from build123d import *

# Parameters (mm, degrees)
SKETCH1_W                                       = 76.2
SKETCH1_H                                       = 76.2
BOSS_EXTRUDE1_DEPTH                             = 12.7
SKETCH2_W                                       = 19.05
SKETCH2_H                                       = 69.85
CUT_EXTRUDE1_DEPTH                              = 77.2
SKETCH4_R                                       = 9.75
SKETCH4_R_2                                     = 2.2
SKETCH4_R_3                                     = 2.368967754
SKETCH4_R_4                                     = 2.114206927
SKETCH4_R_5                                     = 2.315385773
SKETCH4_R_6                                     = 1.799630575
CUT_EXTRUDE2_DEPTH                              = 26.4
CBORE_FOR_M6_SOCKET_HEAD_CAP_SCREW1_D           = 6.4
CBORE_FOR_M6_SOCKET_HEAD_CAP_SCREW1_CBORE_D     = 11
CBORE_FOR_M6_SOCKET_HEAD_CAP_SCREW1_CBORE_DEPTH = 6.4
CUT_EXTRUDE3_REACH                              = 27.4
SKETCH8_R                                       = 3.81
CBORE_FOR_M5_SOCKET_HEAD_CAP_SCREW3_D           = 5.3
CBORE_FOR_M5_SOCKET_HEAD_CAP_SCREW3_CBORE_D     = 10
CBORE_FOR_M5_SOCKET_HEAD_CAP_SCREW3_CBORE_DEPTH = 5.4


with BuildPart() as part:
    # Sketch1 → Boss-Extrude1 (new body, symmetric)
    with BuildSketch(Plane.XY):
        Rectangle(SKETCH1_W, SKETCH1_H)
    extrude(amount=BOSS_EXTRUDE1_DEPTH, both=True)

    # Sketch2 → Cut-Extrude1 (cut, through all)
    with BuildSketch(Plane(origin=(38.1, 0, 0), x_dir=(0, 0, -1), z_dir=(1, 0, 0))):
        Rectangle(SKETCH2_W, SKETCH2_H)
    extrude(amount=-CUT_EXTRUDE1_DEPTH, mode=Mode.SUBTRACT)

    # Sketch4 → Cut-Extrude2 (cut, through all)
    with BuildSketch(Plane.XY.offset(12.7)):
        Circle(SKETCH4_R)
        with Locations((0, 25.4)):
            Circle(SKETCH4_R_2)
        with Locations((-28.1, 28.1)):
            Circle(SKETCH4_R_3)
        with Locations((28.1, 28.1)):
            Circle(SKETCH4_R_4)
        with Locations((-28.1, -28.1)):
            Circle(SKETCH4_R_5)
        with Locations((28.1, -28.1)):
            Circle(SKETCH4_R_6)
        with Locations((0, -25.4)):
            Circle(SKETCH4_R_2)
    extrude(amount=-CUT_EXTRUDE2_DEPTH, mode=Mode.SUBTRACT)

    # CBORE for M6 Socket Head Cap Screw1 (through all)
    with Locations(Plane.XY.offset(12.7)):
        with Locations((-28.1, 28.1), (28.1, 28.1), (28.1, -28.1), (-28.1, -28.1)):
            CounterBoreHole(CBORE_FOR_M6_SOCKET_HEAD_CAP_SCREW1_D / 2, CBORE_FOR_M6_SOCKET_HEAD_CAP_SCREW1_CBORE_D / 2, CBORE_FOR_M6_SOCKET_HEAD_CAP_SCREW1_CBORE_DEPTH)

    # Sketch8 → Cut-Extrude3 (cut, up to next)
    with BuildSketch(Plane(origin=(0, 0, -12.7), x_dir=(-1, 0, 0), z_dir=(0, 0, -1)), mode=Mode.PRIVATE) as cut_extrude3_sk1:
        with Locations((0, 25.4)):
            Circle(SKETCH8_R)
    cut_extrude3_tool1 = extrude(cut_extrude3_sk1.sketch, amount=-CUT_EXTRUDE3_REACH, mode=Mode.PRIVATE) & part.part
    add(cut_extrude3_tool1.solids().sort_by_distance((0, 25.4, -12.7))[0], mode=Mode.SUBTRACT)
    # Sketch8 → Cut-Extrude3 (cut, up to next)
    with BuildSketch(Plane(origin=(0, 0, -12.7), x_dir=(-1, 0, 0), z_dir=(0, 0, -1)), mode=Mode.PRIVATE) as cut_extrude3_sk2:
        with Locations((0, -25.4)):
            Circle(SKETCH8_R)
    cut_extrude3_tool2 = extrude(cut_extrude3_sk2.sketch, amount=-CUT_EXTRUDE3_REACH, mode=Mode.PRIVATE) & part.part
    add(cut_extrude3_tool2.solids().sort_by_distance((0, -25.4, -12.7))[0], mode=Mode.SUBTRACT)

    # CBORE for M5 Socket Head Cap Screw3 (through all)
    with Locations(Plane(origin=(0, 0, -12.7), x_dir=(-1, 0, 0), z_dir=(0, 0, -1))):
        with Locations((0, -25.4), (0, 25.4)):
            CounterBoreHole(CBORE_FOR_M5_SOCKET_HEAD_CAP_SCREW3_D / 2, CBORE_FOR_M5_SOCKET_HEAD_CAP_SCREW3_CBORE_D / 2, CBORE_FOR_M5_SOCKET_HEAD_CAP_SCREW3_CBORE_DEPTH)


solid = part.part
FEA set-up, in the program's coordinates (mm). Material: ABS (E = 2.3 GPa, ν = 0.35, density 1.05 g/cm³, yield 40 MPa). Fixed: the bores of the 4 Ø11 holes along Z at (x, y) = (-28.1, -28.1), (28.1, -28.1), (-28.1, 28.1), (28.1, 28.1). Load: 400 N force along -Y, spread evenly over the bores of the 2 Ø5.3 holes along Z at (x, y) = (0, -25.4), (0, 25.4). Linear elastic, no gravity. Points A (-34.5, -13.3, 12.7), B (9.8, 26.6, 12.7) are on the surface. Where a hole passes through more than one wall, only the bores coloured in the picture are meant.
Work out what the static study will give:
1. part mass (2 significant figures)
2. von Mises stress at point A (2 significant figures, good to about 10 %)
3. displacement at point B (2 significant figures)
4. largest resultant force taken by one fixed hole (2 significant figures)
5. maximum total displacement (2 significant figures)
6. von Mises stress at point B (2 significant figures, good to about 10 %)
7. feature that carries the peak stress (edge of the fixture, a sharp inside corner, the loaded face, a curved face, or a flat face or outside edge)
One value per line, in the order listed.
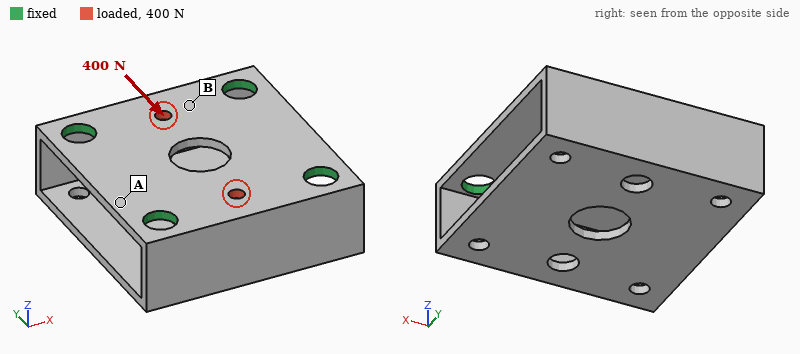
44 g
0.51 MPa
22 µm
100 N
42 µm
1.6 MPa
the loaded face
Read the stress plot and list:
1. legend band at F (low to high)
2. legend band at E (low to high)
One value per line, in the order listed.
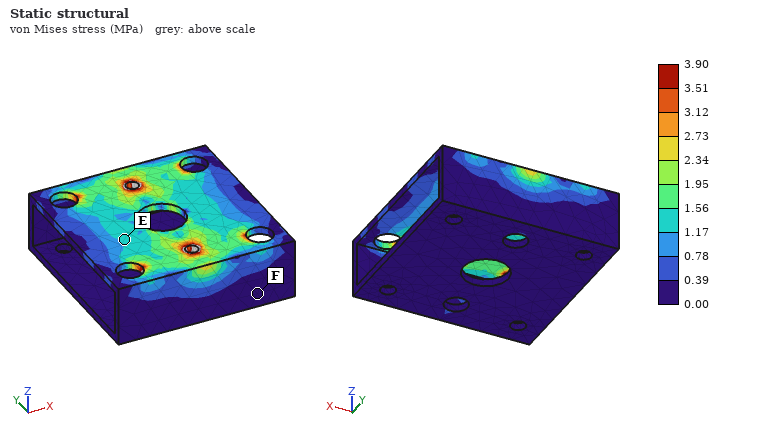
0.00 to 0.39 MPa
1.17 to 1.56 MPa
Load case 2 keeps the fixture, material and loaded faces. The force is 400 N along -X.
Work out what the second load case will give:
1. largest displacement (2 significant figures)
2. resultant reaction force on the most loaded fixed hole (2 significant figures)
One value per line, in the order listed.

20 µm
100 N
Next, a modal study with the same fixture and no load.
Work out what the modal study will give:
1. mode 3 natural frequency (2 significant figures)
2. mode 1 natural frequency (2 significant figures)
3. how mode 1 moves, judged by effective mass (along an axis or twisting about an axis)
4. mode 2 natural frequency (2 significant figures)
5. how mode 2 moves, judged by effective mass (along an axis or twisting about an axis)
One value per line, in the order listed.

880 Hz
640 Hz
along Y
740 Hz
along Z
